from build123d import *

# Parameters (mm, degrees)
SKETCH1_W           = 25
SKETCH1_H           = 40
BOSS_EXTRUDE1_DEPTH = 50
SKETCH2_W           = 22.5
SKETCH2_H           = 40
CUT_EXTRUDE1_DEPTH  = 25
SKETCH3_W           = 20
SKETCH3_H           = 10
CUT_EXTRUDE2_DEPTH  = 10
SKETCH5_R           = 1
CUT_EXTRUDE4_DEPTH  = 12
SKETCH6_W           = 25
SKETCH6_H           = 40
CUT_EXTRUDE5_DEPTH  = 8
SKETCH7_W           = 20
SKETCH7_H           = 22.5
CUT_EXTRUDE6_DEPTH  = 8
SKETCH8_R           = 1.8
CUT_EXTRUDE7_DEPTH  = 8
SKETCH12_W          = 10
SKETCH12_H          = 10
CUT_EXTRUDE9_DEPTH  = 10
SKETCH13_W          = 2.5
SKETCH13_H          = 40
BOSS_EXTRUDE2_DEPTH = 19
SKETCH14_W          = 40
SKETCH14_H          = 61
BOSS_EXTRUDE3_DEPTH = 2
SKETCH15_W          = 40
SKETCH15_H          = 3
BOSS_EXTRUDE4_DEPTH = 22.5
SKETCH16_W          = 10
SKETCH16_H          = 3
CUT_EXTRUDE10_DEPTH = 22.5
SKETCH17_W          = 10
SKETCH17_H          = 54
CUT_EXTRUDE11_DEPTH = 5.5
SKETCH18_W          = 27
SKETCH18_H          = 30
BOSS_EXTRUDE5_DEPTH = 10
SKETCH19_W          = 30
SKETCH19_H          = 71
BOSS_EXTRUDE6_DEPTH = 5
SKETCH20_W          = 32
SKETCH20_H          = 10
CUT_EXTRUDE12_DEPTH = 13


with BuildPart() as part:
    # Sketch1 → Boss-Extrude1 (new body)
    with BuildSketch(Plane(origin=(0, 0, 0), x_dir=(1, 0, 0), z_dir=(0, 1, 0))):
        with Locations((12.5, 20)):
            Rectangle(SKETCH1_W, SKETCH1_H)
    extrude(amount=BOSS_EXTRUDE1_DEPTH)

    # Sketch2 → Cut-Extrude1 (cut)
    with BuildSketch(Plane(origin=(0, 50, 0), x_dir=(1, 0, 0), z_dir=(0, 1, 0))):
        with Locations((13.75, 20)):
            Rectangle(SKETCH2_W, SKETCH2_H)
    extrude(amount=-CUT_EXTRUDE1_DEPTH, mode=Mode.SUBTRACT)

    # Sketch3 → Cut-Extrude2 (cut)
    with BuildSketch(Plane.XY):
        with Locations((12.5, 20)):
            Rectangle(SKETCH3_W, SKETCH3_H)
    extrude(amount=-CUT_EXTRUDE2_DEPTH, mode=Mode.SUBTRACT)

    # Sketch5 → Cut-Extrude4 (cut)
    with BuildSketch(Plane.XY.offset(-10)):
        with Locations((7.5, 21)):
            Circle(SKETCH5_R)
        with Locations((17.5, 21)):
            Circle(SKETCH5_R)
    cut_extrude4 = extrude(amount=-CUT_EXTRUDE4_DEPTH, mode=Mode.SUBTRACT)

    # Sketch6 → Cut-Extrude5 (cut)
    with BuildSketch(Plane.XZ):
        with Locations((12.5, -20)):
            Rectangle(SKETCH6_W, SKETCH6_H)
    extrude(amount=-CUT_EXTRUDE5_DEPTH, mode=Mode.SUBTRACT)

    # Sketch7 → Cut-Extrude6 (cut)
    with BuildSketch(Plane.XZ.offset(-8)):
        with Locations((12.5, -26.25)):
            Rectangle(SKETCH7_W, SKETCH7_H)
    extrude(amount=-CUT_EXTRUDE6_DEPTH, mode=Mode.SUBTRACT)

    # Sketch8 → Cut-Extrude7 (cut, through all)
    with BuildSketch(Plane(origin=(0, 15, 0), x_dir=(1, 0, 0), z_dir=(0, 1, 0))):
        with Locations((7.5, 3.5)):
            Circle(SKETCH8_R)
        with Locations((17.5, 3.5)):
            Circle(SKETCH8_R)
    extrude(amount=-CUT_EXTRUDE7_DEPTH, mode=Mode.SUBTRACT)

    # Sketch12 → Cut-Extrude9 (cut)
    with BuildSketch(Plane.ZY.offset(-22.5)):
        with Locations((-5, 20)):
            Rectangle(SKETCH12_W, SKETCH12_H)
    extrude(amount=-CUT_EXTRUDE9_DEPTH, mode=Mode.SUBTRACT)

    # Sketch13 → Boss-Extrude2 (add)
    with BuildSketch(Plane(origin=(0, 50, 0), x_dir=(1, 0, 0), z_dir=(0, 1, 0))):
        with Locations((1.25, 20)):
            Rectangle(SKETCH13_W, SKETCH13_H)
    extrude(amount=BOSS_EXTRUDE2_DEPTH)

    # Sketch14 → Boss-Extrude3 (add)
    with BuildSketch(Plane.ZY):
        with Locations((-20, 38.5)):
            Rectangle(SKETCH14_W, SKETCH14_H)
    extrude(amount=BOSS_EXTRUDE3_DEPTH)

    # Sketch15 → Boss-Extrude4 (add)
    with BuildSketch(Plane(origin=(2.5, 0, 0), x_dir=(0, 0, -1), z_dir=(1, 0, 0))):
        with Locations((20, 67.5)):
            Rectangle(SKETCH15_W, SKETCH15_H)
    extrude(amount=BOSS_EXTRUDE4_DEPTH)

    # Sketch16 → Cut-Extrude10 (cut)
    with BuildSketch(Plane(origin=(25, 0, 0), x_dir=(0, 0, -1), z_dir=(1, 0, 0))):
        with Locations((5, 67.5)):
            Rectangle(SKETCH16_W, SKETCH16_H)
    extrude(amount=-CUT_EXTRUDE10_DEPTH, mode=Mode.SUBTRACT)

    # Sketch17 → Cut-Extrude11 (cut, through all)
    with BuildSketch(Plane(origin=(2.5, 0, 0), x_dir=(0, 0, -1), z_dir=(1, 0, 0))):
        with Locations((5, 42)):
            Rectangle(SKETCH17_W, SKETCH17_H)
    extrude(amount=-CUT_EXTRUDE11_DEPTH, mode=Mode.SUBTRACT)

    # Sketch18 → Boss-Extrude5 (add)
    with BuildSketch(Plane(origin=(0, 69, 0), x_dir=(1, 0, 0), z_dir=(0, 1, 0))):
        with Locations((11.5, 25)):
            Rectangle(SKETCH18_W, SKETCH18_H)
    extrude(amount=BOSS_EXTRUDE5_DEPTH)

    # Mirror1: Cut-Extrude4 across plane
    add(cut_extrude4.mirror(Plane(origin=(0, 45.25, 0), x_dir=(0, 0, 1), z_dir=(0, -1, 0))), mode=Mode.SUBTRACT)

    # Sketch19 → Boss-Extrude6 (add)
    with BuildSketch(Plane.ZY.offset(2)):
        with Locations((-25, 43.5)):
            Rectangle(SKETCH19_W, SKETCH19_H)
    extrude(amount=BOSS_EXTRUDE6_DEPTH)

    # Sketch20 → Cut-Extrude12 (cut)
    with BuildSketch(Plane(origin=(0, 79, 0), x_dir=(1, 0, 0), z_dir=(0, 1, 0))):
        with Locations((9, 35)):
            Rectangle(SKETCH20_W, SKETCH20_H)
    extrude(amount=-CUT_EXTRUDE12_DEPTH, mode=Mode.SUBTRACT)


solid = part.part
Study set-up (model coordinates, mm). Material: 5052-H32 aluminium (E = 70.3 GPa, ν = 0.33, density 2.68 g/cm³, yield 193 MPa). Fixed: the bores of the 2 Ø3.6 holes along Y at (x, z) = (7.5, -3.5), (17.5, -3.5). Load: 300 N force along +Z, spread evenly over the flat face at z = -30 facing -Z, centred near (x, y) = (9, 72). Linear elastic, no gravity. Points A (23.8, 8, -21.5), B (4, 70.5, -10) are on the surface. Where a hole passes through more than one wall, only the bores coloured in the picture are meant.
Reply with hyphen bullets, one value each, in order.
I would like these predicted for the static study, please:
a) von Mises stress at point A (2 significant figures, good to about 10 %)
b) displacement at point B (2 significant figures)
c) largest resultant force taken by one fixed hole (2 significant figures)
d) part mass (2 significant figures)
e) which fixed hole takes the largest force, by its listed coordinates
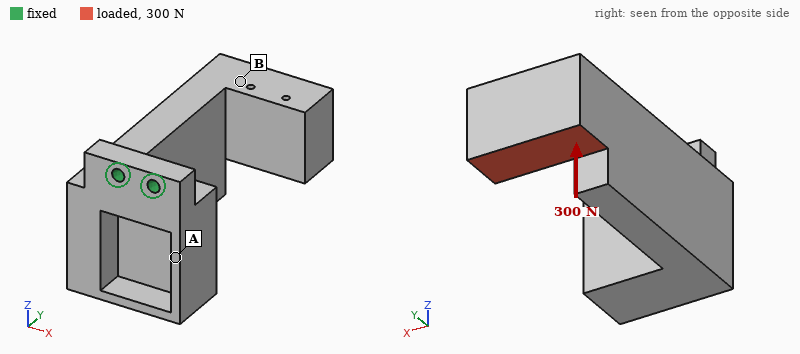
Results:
- 30 MPa
- 0.30 mm
- 340 N
- 92 g
- (7.5, -3.5)
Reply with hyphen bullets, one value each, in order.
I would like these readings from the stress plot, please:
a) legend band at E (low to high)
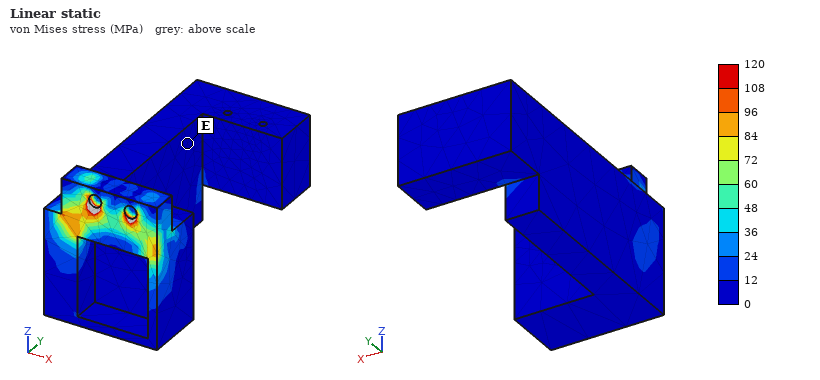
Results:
- 0 to 12 MPa
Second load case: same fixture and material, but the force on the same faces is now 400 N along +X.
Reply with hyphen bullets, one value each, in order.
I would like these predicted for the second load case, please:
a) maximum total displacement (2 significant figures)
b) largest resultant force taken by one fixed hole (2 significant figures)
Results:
- 0.35 mm
- 1.5 kN
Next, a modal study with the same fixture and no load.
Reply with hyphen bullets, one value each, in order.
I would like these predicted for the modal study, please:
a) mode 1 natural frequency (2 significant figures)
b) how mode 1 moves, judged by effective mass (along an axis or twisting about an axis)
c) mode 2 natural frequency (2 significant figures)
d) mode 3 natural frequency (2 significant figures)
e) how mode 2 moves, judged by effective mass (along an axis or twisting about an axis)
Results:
- 790 Hz
- along Z
- 1100 Hz
- 3500 Hz
- along X
